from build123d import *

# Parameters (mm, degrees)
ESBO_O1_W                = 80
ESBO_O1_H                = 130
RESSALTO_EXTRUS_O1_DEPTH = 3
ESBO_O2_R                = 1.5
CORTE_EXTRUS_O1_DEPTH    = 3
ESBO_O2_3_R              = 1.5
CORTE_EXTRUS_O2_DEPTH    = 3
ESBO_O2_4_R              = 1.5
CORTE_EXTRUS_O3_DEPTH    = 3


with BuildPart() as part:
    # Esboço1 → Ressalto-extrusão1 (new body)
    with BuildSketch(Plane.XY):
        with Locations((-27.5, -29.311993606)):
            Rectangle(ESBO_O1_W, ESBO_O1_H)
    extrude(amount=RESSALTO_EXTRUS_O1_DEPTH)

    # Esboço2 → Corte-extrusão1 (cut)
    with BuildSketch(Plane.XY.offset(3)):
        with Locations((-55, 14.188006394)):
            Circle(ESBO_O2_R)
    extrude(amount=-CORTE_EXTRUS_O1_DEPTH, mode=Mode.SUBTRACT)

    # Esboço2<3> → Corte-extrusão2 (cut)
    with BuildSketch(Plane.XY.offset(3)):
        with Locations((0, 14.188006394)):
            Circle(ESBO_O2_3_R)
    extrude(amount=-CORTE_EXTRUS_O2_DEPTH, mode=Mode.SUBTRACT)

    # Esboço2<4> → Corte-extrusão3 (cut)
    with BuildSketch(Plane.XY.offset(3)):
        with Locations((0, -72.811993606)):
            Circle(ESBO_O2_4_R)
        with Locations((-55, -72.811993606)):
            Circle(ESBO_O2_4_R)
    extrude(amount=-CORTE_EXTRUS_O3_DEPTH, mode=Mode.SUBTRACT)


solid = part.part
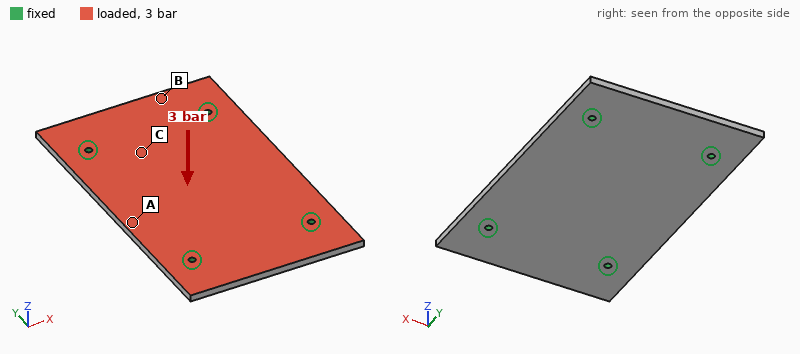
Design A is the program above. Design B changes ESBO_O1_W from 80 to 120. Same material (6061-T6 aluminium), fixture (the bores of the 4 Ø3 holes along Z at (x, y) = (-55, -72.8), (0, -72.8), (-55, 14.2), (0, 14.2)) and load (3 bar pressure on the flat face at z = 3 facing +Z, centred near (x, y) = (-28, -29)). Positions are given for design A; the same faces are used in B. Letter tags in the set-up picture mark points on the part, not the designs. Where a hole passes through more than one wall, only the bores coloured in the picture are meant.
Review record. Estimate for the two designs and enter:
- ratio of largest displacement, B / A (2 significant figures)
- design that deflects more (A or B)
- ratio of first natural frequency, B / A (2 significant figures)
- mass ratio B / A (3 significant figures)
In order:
2.1
B
0.81
1.50
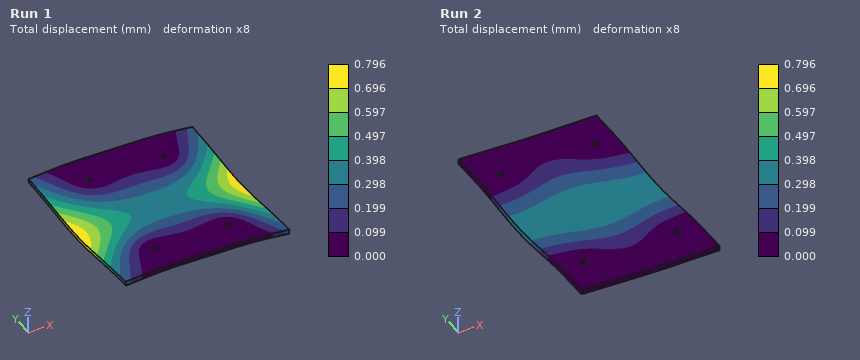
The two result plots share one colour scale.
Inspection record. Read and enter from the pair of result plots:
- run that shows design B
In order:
Run 1
